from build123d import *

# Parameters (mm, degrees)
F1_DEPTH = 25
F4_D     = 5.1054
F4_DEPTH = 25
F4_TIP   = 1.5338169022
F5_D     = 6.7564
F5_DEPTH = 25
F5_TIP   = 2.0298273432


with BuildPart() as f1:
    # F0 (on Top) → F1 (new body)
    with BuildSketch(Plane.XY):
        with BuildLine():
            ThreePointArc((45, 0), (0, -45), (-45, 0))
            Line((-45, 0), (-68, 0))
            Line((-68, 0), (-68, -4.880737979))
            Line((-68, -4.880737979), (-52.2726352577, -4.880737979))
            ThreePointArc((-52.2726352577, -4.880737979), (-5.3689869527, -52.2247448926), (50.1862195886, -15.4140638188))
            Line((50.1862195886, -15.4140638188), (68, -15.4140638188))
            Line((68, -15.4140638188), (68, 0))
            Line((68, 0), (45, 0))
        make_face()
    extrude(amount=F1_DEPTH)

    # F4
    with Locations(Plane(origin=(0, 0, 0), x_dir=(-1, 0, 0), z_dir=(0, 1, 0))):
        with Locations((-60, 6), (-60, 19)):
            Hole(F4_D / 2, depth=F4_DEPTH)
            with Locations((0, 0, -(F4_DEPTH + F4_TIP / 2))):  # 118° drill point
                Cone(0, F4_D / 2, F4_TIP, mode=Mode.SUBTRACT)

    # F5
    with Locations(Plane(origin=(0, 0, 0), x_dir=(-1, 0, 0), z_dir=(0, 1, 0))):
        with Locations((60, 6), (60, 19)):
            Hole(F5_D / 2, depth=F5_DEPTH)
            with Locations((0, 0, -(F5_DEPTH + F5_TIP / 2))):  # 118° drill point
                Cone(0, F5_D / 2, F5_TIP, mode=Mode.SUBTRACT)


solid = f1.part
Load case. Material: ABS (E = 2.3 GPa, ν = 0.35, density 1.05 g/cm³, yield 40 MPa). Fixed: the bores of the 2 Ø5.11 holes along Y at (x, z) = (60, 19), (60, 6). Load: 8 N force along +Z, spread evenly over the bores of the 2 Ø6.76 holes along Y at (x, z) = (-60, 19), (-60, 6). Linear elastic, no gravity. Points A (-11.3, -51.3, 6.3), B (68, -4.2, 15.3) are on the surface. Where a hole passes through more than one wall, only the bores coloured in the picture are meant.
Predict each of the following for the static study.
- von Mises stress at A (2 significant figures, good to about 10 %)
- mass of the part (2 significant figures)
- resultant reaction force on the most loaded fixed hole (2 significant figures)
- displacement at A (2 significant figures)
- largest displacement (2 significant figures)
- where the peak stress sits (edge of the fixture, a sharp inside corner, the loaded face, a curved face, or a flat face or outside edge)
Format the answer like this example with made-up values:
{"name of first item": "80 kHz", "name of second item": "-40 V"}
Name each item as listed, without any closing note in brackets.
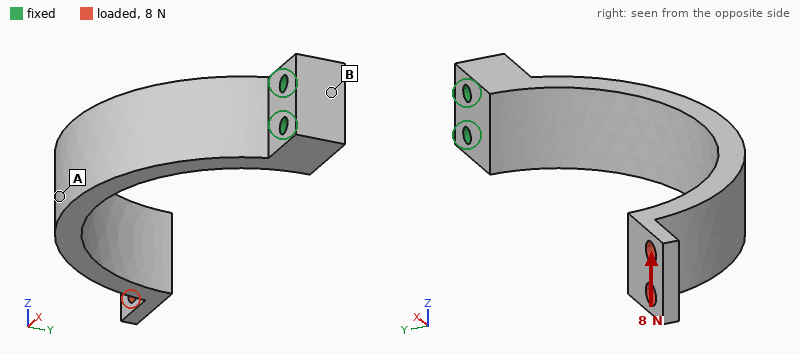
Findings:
{"von Mises stress at A": "0.99 MPa", "mass of the part": "38 g", "resultant reaction force on the most loaded fixed hole": "61 N", "displacement at A": "0.35 mm", "largest displacement": "1.7 mm", "where the peak stress sits": "a curved face"}
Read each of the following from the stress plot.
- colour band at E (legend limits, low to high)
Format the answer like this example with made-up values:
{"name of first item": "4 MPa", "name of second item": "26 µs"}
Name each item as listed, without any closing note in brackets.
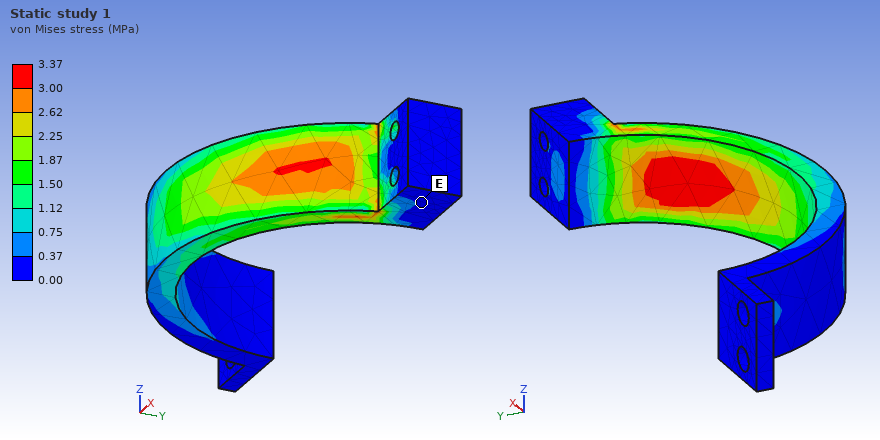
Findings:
{"colour band at E": "0.00 to 0.37 MPa"}
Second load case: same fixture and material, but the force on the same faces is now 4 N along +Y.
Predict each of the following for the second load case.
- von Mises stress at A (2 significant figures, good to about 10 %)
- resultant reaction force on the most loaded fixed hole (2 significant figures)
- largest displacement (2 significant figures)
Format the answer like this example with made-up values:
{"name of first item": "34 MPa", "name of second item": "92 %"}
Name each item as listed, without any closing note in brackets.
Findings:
{"von Mises stress at A": "0.79 MPa", "resultant reaction force on the most loaded fixed hole": "5.0 N", "largest displacement": "1.5 mm"}
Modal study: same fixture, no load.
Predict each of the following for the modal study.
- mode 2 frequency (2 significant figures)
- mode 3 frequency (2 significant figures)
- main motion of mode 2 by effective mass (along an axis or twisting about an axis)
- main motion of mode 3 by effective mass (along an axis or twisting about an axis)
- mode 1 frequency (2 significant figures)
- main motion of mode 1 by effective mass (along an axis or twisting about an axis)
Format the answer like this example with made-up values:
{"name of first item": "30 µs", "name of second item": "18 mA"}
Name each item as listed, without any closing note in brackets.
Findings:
{"mode 2 frequency": "140 Hz", "mode 3 frequency": "310 Hz", "main motion of mode 2 by effective mass": "along Z", "main motion of mode 3 by effective mass": "along X", "mode 1 frequency": "94 Hz", "main motion of mode 1 by effective mass": "along Y"}
